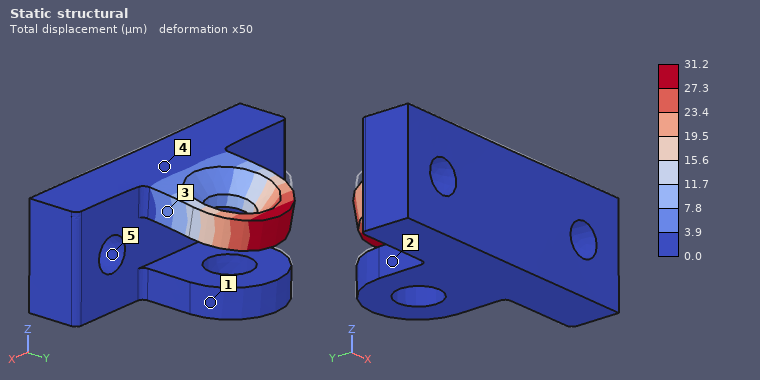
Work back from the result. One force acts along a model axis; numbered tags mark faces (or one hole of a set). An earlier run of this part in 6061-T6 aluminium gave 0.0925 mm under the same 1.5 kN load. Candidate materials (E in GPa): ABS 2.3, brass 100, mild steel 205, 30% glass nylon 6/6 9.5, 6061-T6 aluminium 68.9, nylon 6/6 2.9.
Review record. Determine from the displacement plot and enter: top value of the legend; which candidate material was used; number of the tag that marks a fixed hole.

31.2 µm
mild steel
5
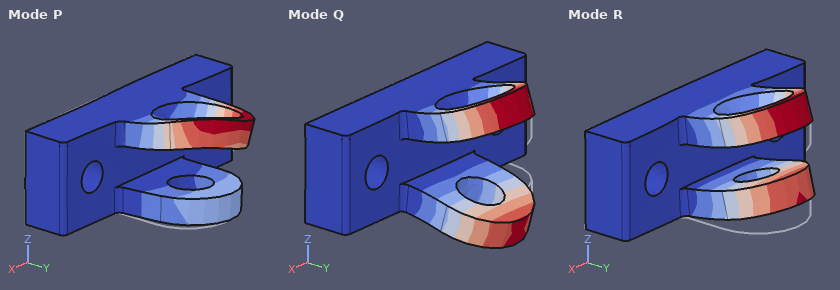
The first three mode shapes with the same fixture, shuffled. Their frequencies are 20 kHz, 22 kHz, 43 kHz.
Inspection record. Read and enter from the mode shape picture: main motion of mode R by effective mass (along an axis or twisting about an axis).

along Z
